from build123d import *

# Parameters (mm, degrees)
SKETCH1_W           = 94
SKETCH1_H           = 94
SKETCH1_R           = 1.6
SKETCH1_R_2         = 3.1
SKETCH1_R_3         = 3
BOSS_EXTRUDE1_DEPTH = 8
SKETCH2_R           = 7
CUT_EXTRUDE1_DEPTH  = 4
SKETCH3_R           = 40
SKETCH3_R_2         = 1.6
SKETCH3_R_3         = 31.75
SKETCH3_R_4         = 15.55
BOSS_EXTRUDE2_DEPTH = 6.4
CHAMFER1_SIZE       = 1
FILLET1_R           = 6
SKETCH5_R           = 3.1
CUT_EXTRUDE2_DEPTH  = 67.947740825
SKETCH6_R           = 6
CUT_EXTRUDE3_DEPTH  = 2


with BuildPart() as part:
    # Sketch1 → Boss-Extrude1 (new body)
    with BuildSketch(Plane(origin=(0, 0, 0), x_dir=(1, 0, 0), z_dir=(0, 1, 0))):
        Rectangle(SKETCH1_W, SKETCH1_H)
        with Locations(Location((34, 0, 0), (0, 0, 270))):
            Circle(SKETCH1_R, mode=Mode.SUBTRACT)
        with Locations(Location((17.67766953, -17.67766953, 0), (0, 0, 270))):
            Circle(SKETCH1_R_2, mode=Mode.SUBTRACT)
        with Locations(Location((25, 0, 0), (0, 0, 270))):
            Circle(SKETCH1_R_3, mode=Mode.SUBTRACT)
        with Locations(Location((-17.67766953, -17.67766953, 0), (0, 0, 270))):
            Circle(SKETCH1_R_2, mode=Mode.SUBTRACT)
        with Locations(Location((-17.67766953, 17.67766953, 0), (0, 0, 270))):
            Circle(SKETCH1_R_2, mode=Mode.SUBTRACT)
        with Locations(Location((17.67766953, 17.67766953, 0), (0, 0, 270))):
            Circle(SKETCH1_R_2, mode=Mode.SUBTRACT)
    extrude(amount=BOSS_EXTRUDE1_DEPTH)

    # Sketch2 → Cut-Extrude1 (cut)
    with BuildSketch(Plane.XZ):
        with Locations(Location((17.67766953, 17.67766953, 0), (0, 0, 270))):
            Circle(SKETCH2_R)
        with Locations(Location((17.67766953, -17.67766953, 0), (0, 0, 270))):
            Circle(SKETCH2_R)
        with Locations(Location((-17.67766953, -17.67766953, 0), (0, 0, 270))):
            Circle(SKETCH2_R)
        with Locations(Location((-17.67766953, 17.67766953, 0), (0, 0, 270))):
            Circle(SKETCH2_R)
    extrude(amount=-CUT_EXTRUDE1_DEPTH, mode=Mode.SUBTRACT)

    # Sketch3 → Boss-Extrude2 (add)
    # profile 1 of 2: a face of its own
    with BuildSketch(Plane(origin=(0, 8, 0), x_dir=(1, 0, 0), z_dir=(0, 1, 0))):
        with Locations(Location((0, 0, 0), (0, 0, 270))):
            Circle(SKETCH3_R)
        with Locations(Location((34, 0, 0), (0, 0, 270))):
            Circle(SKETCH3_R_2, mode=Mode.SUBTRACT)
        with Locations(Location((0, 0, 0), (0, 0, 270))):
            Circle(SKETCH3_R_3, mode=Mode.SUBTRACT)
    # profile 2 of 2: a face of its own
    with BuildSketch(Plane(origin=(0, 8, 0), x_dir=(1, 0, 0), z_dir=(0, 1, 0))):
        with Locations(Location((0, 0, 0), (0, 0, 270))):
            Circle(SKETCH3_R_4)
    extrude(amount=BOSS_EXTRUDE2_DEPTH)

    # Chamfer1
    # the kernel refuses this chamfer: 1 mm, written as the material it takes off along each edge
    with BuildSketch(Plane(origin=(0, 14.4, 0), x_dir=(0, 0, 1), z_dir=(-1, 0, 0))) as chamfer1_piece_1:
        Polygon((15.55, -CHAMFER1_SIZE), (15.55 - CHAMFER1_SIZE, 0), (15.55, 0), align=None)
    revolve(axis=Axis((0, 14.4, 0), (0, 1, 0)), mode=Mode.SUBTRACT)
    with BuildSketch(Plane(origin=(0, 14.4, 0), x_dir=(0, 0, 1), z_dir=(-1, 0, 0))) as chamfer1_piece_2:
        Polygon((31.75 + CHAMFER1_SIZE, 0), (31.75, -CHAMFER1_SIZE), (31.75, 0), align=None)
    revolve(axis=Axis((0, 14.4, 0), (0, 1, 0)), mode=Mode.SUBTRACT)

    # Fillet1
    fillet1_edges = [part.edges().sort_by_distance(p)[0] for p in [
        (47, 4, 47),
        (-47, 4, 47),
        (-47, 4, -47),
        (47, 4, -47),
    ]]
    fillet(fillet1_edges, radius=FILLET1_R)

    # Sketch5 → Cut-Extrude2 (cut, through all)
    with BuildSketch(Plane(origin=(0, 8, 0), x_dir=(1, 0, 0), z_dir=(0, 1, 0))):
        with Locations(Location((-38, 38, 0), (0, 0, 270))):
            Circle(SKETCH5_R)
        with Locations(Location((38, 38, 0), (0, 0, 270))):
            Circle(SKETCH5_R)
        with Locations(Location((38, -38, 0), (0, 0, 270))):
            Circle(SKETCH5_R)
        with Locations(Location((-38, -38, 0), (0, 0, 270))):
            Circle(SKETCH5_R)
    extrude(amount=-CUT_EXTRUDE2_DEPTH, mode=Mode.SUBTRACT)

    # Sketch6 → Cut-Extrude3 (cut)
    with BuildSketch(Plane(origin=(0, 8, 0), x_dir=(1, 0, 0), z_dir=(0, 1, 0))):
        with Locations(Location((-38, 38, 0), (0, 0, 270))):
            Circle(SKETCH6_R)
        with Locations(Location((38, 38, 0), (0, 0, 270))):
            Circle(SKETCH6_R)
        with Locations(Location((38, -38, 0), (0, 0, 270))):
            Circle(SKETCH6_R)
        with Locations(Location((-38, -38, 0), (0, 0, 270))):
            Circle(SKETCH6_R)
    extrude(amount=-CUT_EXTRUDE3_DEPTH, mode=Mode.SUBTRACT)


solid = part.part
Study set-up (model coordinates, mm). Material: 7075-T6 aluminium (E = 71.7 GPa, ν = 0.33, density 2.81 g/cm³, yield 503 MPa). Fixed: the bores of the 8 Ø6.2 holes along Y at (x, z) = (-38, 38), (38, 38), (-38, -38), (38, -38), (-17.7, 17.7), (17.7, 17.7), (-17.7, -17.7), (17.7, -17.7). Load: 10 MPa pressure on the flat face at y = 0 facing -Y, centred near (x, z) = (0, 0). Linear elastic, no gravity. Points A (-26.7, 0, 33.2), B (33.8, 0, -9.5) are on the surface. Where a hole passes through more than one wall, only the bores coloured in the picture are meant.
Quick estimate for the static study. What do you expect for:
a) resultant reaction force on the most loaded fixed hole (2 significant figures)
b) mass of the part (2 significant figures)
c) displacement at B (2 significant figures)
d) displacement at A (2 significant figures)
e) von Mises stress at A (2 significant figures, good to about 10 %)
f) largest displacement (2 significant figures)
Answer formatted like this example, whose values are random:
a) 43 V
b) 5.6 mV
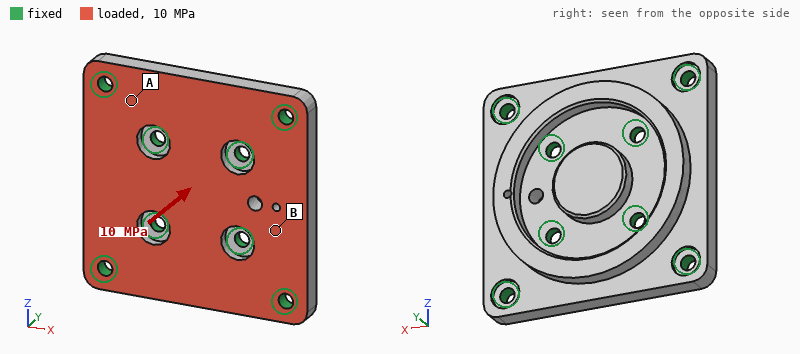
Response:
a) 12 kN
b) 230 g
c) 0.069 mm
d) 0.036 mm
e) 110 MPa
f) 0.12 mm
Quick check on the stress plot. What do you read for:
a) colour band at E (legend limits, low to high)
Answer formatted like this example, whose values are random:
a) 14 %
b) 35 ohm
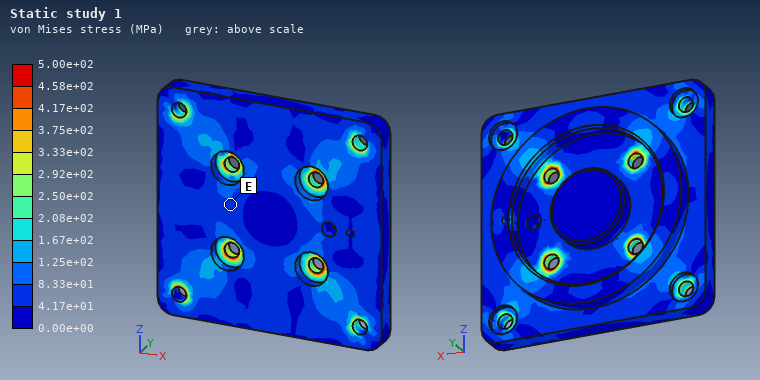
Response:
a) 4.17e+01 to 8.33e+01 MPa
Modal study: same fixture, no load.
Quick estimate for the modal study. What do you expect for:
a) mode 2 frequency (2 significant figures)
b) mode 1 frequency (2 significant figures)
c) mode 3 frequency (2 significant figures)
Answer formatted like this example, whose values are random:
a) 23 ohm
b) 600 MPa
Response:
a) 10 kHz
b) 8500 Hz
c) 10 kHz
